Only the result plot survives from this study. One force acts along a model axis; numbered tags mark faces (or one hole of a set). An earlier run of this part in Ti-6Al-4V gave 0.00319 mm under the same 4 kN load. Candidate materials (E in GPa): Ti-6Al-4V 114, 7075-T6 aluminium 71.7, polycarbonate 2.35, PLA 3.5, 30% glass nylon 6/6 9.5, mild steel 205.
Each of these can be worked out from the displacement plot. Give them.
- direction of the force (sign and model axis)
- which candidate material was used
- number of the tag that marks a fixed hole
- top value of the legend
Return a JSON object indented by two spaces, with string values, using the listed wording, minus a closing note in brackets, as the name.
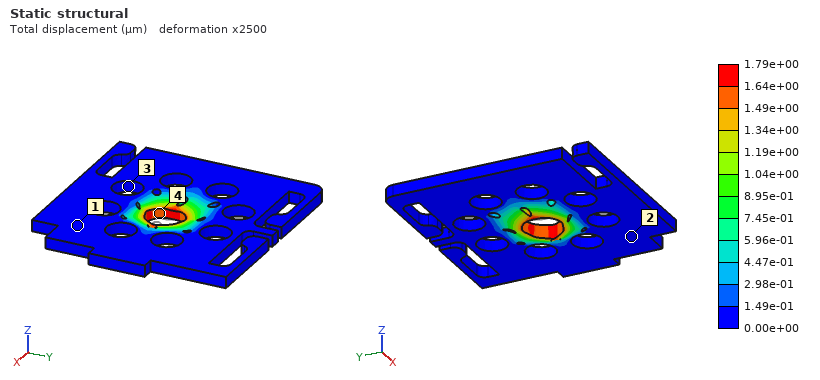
{
  "direction of the force": "+X",
  "which candidate material was used": "mild steel",
  "number of the tag that marks a fixed hole": "3",
  "top value of the legend": "1.79e+00 µm"
}
